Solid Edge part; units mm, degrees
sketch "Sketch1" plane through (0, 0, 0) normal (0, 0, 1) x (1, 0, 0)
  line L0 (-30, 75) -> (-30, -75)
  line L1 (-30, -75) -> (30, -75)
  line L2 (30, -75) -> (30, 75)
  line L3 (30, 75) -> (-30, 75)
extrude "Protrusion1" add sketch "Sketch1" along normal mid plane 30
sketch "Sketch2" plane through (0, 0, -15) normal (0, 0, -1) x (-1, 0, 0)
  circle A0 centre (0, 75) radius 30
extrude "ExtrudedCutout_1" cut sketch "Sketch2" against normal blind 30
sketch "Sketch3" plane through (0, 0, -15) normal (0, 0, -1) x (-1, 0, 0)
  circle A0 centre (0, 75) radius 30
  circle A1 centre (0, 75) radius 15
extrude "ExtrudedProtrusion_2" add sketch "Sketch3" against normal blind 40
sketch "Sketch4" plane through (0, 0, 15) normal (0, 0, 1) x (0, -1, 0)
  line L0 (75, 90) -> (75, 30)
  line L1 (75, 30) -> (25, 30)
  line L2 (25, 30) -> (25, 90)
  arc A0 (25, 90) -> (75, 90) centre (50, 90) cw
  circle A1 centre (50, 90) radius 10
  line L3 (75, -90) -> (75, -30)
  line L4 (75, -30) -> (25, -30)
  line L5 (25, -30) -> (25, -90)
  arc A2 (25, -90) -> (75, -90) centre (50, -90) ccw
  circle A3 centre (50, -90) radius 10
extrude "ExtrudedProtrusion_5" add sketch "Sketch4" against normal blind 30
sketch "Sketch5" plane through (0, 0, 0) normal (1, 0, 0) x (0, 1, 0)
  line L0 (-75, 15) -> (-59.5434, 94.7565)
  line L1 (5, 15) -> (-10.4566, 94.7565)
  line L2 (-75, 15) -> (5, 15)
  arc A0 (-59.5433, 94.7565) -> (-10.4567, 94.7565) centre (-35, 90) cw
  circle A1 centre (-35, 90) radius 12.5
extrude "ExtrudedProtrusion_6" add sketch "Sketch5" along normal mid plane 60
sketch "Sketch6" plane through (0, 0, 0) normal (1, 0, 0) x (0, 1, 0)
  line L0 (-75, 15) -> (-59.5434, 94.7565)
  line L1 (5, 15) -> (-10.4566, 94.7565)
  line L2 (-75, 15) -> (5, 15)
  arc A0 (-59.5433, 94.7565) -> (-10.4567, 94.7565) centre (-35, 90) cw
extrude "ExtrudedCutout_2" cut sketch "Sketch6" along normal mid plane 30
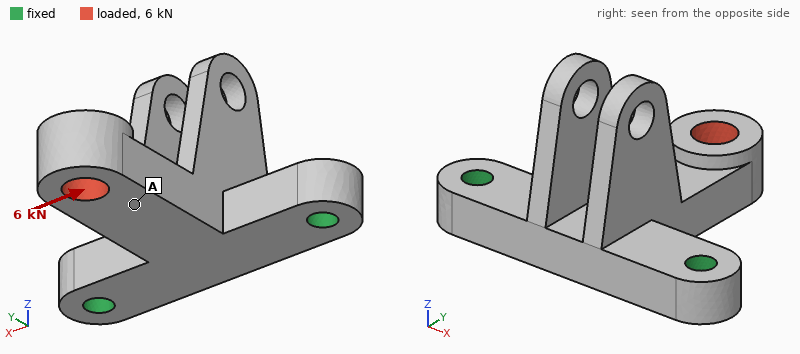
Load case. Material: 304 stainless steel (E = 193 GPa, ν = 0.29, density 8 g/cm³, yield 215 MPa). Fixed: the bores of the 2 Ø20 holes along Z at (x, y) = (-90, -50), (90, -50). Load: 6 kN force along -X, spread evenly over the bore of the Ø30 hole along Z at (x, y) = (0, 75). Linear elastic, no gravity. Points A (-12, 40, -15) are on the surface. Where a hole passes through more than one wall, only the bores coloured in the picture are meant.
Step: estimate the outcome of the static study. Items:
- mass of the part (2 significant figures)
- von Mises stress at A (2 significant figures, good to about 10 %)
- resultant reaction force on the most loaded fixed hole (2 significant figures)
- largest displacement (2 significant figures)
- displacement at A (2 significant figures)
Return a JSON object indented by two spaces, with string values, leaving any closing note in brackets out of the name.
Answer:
{
  "mass of the part": "5.6 kg",
  "von Mises stress at A": "5.4 MPa",
  "resultant reaction force on the most loaded fixed hole": "6.0 kN",
  "largest displacement": "60 µm",
  "displacement at A": "25 µm"
}
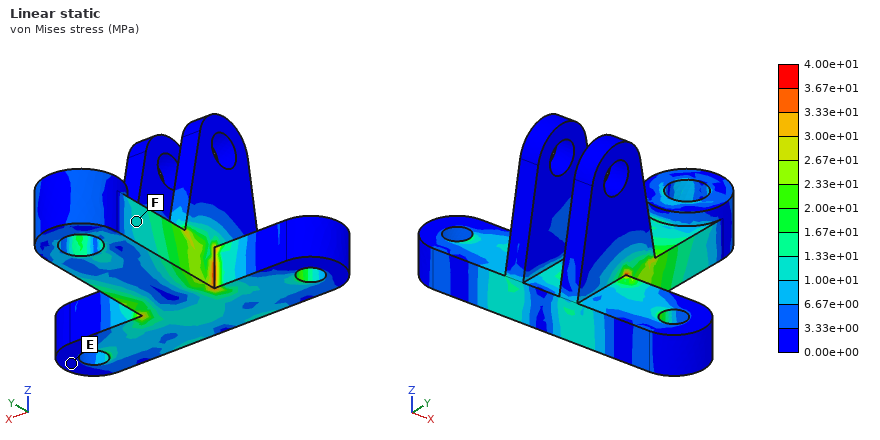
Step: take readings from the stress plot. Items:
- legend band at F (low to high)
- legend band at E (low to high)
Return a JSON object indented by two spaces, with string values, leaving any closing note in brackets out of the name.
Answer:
{
  "legend band at F": "1.00e+01 to 1.33e+01 MPa",
  "legend band at E": "0.00e+00 to 3.33e+00 MPa"
}
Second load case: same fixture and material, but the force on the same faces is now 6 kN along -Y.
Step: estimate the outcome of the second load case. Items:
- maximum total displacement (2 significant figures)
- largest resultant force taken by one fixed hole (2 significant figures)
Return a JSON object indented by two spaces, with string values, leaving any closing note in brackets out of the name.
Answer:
{
  "maximum total displacement": "17 µm",
  "largest resultant force taken by one fixed hole": "3.1 kN"
}
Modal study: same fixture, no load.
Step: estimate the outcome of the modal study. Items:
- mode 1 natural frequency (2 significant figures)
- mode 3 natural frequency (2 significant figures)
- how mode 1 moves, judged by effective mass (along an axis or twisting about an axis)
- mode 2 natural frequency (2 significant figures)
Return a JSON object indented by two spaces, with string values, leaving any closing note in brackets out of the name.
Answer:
{
  "mode 1 natural frequency": "780 Hz",
  "mode 3 natural frequency": "1500 Hz",
  "how mode 1 moves, judged by effective mass": "along Z",
  "mode 2 natural frequency": "1500 Hz"
}
